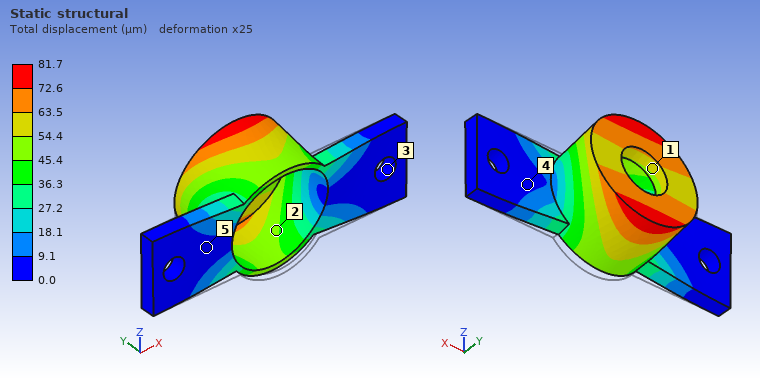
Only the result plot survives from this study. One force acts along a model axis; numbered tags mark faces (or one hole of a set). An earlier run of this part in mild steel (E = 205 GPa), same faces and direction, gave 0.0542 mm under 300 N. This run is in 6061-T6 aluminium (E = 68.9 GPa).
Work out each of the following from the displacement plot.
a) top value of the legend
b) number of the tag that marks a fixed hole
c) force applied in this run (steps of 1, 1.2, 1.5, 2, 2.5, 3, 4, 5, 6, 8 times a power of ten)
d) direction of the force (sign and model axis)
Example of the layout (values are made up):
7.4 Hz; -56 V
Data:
81.7 µm; 3; 150 N; +Z
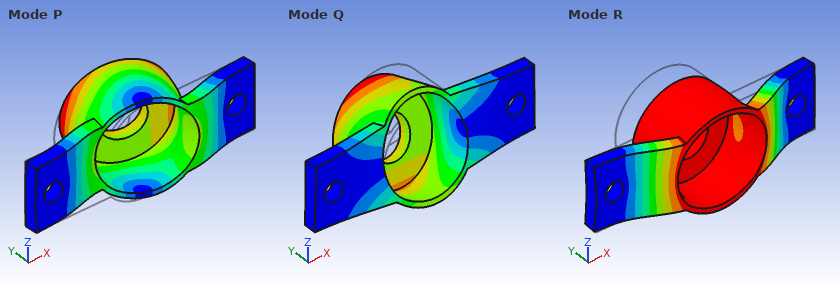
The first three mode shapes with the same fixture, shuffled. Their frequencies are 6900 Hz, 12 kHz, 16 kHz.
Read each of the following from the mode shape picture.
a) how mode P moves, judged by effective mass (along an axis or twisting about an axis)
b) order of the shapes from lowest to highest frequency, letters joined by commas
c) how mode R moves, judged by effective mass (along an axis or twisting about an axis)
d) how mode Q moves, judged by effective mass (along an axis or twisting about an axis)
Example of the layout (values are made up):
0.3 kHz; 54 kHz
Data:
along X; Q, R, P; along Y; along Z
